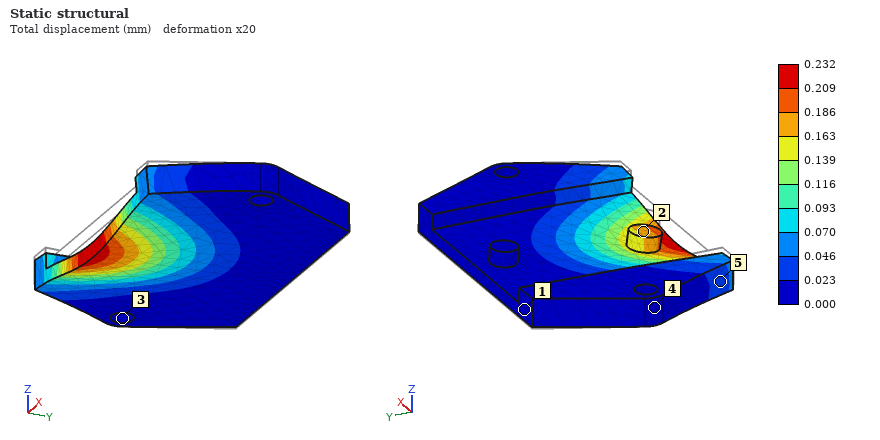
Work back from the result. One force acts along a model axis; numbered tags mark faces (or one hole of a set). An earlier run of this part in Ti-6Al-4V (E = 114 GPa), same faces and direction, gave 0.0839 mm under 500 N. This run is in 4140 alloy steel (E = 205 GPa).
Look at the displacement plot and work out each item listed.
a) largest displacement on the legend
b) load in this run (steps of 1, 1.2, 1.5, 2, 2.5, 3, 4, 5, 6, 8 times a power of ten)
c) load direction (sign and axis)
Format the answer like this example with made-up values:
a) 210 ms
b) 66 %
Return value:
a) 0.232 mm
b) 2.5 kN
c) -Z
